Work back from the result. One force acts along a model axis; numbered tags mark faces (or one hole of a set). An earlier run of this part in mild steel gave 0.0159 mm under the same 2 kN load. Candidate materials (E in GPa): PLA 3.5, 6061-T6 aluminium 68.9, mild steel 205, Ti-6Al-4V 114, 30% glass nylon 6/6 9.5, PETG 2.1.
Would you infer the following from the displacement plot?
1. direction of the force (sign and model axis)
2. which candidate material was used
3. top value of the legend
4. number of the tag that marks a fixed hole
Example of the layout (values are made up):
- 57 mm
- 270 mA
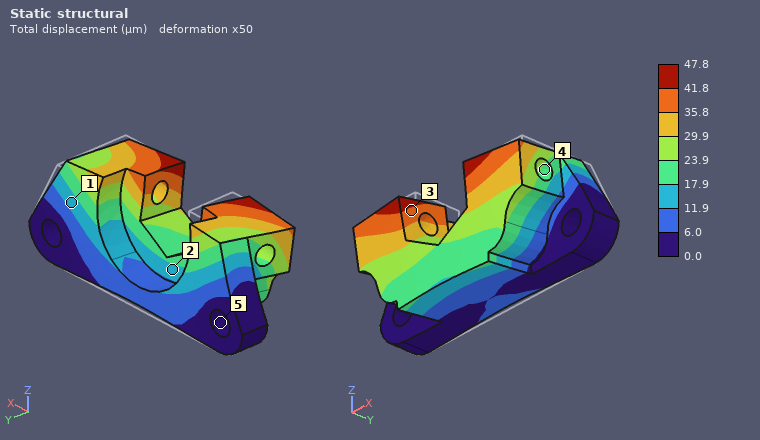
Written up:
- -Y
- 6061-T6 aluminium
- 47.8 µm
- 5
